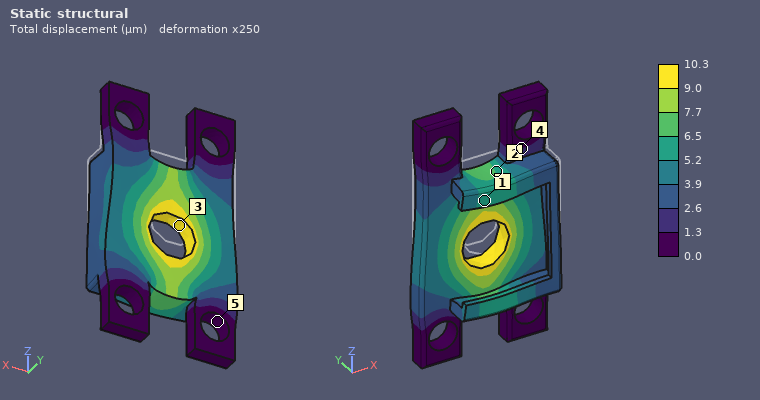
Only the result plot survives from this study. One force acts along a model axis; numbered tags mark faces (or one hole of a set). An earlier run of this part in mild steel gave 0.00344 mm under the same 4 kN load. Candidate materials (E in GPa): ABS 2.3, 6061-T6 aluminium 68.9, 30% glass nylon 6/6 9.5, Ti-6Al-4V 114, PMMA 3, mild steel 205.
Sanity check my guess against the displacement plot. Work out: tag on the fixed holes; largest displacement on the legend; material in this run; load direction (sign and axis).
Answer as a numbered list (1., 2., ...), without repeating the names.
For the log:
1. 5
2. 10.3 µm
3. 6061-T6 aluminium
4. -Z
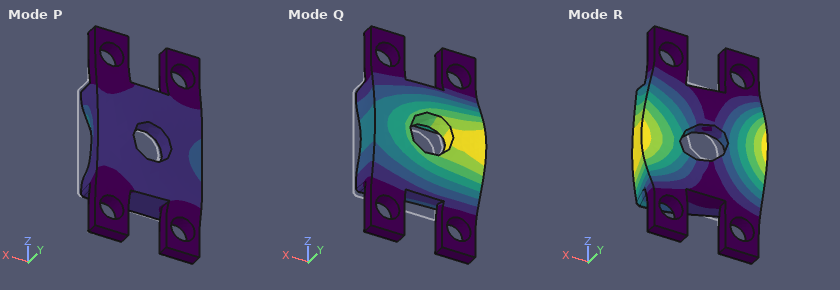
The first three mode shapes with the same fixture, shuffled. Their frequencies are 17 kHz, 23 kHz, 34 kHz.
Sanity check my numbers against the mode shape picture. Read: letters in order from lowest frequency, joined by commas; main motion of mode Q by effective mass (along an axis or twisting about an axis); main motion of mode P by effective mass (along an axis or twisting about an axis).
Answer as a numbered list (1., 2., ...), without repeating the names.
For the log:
1. Q, R, P
2. along Y
3. along X
